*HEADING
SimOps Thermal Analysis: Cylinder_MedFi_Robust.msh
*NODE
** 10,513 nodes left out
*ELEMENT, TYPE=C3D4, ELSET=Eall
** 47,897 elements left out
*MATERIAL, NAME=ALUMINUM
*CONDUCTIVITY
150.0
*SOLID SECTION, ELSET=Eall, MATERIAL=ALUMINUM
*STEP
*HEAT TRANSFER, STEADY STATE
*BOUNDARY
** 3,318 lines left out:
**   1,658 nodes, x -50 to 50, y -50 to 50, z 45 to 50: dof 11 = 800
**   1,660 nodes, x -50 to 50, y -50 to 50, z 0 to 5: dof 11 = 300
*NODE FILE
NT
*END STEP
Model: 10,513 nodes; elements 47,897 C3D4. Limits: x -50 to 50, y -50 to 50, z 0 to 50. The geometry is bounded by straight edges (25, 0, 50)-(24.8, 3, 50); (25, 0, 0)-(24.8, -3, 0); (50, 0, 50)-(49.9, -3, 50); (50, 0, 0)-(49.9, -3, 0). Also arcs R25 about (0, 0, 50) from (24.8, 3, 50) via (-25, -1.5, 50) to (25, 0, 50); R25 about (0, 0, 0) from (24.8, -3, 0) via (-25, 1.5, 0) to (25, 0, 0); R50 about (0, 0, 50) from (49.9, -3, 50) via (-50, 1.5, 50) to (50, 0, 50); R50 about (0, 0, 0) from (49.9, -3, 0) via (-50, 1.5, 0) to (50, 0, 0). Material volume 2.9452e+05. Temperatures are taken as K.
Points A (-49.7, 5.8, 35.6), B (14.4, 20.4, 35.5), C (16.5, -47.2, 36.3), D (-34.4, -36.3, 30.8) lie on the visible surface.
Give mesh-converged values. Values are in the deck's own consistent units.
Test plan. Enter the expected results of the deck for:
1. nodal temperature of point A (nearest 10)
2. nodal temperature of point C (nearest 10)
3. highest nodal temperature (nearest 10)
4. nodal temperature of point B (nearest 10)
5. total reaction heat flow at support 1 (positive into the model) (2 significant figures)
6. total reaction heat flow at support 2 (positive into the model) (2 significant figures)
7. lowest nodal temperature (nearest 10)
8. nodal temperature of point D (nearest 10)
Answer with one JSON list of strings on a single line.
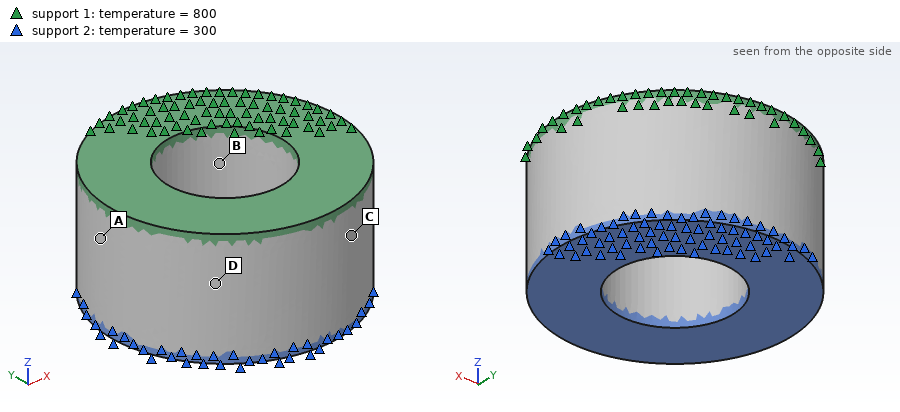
["670 K", "680 K", "800 K", "670 K", "1.0e+07", "-1.0e+07", "300 K", "620 K"]
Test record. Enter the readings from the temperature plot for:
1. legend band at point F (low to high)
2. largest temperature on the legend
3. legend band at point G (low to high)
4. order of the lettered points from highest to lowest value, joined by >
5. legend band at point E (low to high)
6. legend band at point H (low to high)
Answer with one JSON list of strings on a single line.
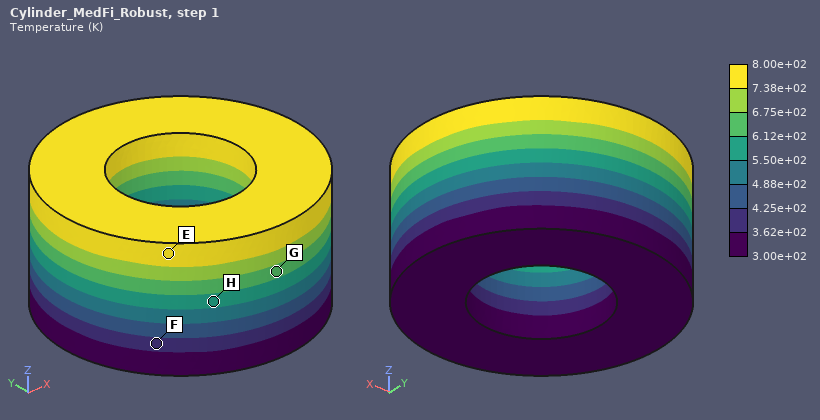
["3.62e+02 to 4.25e+02 K", "8.00e+02 K", "6.12e+02 to 6.75e+02 K", "E > G > H > F", "7.38e+02 to 8.00e+02 K", "5.50e+02 to 6.12e+02 K"]
